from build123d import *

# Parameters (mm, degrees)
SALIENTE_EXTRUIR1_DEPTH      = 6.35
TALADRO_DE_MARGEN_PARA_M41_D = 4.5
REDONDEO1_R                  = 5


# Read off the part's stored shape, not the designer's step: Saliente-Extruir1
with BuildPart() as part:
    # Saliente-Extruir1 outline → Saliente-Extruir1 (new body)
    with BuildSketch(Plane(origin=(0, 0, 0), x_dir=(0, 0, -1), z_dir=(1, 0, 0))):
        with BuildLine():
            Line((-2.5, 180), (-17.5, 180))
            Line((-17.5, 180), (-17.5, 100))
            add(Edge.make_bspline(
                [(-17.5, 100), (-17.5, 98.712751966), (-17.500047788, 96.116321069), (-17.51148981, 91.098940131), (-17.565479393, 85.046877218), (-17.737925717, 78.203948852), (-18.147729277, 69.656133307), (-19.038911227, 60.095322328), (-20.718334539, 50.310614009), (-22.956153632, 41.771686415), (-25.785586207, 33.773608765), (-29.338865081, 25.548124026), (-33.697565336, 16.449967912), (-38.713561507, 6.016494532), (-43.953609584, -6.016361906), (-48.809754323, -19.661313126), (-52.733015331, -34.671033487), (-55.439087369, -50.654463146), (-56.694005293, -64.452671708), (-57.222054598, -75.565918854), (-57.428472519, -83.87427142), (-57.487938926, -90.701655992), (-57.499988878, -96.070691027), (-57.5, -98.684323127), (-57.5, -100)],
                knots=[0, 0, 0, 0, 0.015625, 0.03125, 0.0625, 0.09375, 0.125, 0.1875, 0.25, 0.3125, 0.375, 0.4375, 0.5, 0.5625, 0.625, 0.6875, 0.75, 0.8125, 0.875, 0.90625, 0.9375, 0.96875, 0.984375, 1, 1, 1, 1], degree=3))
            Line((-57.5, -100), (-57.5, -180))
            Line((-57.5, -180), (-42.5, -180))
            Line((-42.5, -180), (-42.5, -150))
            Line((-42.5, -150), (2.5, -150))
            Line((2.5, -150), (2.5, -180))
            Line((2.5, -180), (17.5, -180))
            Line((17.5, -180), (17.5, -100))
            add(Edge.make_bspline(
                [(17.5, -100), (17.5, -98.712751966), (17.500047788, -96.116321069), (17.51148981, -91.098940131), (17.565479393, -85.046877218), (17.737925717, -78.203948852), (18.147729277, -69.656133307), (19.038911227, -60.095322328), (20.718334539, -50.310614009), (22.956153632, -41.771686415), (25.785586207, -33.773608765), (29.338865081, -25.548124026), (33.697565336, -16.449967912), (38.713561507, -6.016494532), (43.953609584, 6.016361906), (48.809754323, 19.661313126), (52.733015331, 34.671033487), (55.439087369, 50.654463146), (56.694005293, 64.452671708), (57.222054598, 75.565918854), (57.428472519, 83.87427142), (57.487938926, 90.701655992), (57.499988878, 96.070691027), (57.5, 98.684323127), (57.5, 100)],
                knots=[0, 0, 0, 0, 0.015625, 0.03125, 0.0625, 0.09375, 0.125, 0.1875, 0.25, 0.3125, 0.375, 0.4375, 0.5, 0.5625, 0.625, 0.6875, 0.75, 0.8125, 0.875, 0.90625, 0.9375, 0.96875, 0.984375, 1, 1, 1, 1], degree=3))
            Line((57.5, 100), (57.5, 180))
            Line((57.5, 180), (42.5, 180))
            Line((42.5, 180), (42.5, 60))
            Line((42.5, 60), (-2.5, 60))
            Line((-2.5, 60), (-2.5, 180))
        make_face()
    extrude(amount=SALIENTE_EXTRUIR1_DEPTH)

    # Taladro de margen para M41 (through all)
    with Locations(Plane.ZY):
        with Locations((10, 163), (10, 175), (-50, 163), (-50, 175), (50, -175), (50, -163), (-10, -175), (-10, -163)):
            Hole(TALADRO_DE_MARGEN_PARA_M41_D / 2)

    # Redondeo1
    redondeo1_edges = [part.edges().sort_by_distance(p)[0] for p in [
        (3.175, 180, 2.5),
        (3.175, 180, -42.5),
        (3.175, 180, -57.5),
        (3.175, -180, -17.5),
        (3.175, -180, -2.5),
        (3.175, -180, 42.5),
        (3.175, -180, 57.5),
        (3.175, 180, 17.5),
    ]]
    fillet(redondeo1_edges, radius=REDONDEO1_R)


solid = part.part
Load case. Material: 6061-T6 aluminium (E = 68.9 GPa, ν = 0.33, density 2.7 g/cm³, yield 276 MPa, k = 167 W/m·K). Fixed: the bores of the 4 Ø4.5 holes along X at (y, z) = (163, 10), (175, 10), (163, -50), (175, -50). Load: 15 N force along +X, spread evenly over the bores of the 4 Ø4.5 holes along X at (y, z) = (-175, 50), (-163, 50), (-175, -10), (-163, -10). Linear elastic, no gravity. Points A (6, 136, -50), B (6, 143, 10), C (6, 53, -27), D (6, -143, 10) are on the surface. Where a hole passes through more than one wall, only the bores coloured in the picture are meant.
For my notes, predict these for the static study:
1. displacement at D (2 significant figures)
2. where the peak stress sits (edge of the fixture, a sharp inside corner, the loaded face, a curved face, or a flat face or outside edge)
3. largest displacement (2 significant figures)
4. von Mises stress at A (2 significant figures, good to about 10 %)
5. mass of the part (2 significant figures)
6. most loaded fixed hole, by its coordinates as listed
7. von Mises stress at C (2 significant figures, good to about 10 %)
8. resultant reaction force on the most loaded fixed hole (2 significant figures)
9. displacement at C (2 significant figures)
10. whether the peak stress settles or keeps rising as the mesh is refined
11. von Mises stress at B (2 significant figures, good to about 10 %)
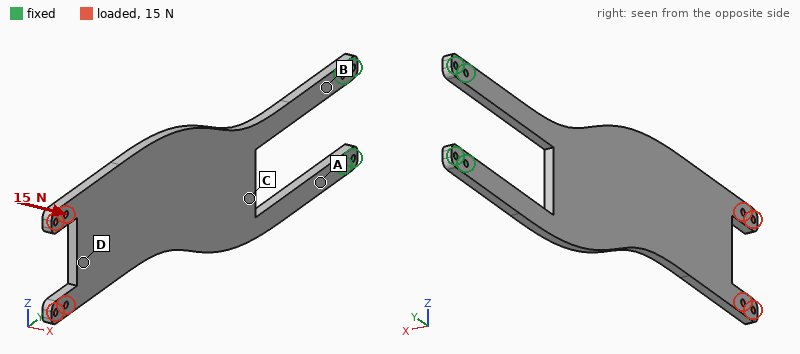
3.1 mm
edge of the fixture
3.7 mm
21 MPa
350 g
(163, 10)
4.8 MPa
55 N
0.60 mm
keeps rising
25 MPa
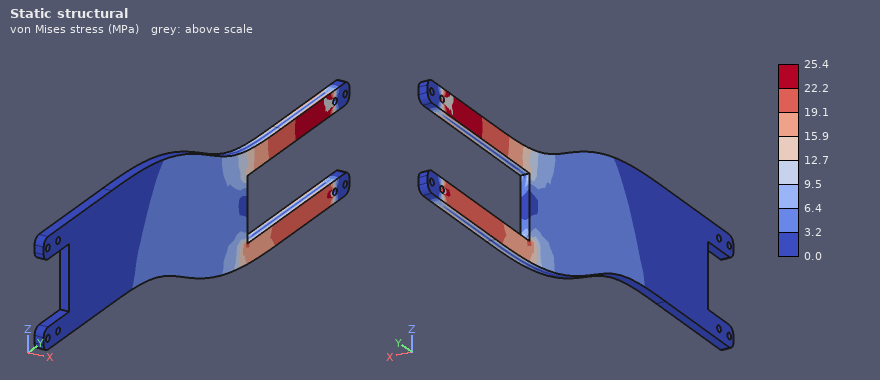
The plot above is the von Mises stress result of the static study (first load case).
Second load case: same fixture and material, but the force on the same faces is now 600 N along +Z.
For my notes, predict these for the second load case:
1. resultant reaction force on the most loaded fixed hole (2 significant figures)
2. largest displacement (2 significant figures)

2.6 kN
0.97 mm
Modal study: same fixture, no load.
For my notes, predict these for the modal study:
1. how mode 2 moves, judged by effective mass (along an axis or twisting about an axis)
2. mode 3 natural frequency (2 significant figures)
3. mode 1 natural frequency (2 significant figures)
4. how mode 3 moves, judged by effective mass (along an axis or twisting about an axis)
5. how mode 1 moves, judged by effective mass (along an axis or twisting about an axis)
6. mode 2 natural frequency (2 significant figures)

along X
280 Hz
32 Hz
twisting about Y
along X
260 Hz
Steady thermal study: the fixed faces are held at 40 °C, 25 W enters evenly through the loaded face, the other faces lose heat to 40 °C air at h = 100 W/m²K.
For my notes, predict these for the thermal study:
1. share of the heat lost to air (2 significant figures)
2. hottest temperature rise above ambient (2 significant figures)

99 %
32 K
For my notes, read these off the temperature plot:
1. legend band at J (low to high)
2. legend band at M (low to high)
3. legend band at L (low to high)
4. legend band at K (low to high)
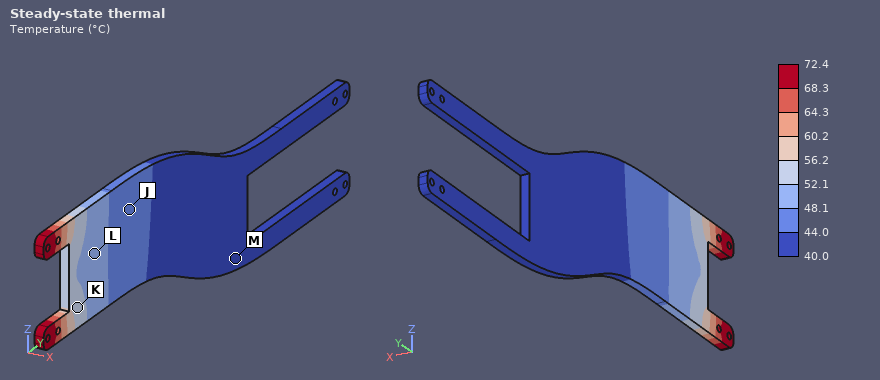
44.0 to 48.1 °C
40.0 to 44.0 °C
48.1 to 52.1 °C
52.1 to 56.2 °C
